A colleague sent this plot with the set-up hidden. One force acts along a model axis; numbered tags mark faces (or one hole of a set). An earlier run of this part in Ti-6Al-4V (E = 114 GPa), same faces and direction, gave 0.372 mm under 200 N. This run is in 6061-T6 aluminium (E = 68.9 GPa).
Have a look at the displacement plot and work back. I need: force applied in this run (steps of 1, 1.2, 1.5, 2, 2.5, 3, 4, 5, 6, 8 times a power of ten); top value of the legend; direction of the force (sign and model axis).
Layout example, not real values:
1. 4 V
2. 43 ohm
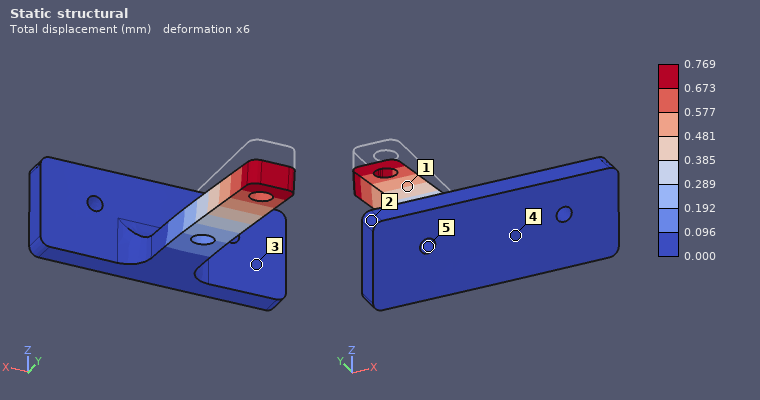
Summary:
1. 250 N
2. 0.769 mm
3. -Z
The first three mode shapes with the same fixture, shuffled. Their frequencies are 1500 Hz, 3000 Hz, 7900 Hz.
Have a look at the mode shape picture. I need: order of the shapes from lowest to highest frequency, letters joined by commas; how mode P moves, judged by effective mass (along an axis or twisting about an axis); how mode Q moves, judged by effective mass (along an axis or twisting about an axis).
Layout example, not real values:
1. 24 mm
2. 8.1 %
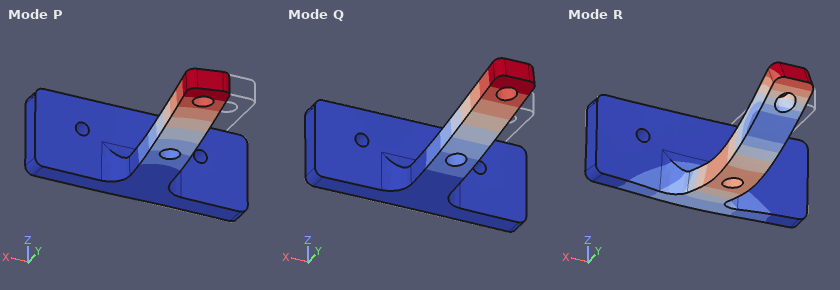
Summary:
1. Q, P, R
2. along X
3. along Z
